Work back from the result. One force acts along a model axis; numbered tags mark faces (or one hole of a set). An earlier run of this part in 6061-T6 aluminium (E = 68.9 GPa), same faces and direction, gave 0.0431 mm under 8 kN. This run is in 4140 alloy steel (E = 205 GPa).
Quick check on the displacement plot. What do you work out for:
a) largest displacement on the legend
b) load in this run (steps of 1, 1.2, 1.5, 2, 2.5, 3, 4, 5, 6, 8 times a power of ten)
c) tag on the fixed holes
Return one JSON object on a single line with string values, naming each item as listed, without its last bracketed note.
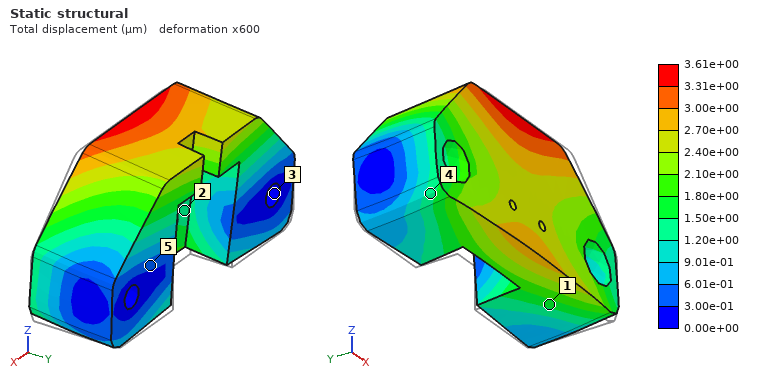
{"largest displacement on the legend": "3.61e+00 µm", "load in this run": "2 kN", "tag on the fixed holes": "3"}
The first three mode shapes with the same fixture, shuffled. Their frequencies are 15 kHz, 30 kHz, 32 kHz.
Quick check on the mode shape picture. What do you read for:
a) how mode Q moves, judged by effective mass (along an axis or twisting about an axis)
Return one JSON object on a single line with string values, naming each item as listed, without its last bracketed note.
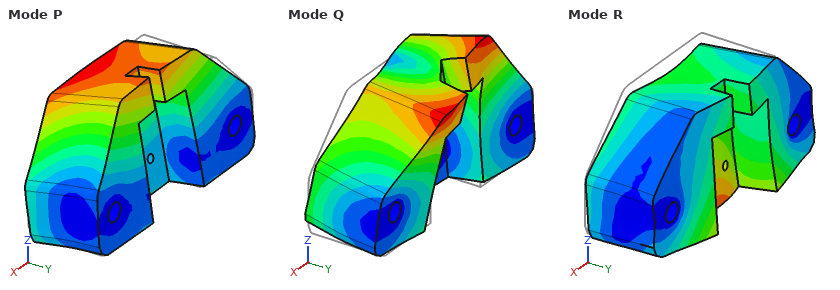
{"how mode Q moves, judged by effective mass": "along X"}
